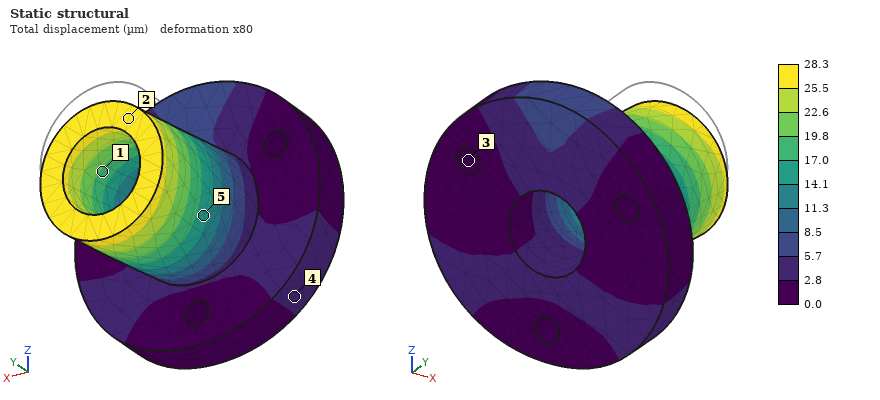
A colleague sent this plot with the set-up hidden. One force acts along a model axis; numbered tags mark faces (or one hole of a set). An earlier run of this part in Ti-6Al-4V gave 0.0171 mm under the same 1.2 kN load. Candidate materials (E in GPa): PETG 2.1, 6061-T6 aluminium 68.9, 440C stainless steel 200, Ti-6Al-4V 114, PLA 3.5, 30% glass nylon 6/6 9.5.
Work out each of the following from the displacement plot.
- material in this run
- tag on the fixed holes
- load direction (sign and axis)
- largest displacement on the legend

6061-T6 aluminium
3
-Z
28.3 µm
